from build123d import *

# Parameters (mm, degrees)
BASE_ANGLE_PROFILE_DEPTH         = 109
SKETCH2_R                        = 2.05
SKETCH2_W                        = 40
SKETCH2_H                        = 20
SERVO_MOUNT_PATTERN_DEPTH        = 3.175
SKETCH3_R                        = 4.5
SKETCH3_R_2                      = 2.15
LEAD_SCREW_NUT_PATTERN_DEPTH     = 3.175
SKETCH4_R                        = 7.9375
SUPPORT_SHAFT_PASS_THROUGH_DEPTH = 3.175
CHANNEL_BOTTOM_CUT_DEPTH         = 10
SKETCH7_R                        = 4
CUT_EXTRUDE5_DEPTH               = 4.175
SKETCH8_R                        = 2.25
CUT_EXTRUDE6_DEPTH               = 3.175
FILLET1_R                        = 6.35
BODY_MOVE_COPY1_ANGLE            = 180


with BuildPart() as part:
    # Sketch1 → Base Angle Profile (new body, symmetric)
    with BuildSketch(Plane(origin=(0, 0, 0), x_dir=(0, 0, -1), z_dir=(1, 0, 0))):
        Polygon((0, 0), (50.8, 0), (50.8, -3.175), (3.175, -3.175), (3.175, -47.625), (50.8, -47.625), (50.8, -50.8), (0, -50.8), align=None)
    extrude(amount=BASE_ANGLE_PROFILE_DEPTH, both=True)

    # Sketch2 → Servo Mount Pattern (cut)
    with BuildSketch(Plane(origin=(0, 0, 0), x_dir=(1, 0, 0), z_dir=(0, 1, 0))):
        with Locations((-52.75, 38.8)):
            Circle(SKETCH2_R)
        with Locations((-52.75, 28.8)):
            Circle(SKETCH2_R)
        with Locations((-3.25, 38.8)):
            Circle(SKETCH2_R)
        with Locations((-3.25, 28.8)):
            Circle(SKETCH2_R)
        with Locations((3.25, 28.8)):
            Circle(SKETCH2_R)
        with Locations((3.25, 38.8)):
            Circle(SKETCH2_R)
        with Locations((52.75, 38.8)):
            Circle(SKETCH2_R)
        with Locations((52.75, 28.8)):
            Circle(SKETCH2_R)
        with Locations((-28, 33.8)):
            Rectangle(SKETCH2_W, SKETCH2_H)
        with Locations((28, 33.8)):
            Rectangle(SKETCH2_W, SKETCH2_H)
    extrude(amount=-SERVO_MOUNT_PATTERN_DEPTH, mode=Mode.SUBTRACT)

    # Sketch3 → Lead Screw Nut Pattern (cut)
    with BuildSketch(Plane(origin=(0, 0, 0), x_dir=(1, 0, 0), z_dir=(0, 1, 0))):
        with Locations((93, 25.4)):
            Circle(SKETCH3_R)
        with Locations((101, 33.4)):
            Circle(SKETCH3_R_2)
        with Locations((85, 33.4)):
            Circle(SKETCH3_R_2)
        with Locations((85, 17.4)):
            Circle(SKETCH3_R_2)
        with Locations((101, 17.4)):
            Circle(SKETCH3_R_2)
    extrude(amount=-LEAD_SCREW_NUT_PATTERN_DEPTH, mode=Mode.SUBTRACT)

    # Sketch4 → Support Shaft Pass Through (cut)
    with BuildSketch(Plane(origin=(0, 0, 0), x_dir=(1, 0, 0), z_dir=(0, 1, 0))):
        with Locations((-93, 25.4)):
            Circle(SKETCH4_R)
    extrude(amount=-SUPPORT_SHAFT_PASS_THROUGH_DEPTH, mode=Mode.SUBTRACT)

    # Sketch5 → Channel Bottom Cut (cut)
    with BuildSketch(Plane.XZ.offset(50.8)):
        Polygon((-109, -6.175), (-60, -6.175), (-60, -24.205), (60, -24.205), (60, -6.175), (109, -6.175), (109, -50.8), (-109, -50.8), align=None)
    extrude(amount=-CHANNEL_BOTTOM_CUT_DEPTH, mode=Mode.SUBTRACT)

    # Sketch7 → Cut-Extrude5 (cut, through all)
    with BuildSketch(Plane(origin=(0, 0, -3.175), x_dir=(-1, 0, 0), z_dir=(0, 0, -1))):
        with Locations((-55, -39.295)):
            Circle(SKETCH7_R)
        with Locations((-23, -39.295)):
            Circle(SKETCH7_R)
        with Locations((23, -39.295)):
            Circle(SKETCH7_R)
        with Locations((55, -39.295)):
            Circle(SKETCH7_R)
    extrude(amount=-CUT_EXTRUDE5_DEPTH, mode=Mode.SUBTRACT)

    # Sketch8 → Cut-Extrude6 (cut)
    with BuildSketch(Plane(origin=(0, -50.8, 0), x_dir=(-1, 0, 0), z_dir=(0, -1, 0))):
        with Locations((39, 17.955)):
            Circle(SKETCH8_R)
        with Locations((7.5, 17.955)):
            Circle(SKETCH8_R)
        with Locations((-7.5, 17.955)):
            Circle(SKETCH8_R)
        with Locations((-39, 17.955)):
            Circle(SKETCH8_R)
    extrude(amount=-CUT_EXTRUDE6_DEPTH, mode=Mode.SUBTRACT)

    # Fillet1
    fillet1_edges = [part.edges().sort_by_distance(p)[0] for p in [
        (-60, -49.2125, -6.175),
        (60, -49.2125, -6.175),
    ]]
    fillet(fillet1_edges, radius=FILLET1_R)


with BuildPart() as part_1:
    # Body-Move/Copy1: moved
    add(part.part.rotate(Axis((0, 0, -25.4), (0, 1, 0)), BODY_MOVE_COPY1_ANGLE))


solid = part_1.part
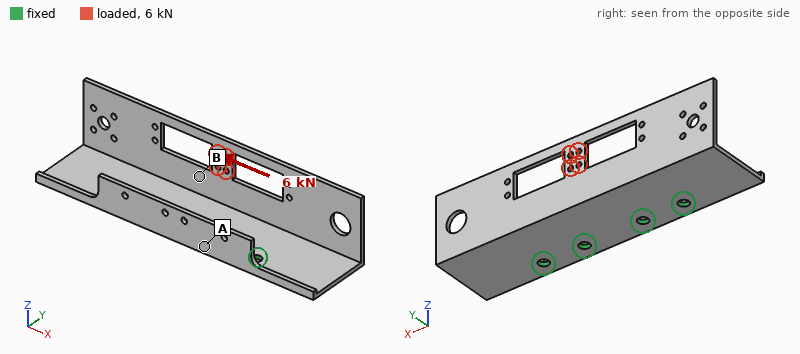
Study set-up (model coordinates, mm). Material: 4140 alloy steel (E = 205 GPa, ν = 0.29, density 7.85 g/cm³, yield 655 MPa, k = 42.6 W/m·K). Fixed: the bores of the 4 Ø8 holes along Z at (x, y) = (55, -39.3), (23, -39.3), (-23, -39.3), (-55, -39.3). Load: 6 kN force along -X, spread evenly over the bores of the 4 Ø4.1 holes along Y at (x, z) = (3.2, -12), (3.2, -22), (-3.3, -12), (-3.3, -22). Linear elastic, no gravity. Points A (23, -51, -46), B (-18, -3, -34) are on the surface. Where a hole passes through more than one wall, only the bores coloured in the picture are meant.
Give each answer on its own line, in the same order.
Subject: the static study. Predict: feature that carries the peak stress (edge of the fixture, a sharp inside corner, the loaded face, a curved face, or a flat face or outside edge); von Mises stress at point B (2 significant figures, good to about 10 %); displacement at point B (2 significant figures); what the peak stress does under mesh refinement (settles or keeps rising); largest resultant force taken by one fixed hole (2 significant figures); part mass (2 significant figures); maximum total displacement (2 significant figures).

edge of the fixture
180 MPa
0.23 mm
keeps rising
2.7 kN
550 g
1.4 mm
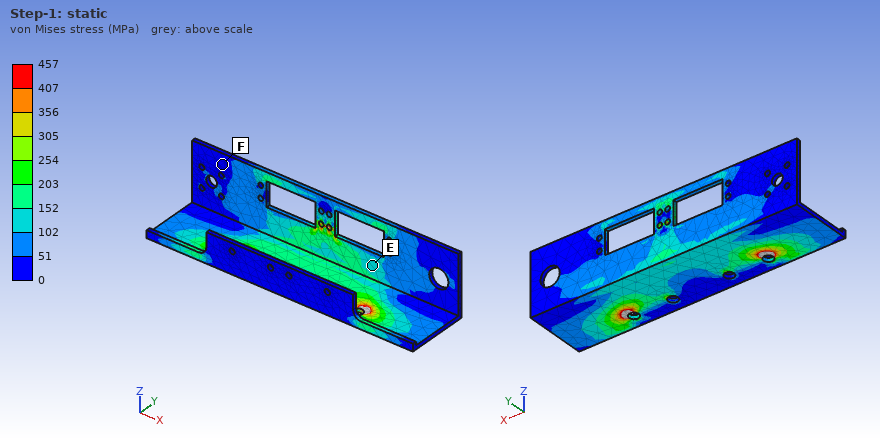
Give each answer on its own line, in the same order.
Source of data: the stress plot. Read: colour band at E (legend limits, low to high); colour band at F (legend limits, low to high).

102 to 152 MPa
0 to 51 MPa
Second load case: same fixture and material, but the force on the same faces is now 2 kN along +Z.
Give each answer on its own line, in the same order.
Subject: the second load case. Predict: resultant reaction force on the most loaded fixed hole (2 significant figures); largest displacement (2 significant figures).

770 N
0.74 mm
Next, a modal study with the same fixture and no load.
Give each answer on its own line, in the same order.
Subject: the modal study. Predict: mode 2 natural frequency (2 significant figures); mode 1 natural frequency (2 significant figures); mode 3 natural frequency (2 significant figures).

520 Hz
500 Hz
1000 Hz
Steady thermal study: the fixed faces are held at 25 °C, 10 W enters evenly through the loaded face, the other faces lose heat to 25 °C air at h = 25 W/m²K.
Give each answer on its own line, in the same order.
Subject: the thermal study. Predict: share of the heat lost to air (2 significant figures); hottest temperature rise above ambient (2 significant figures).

67 %
67 K
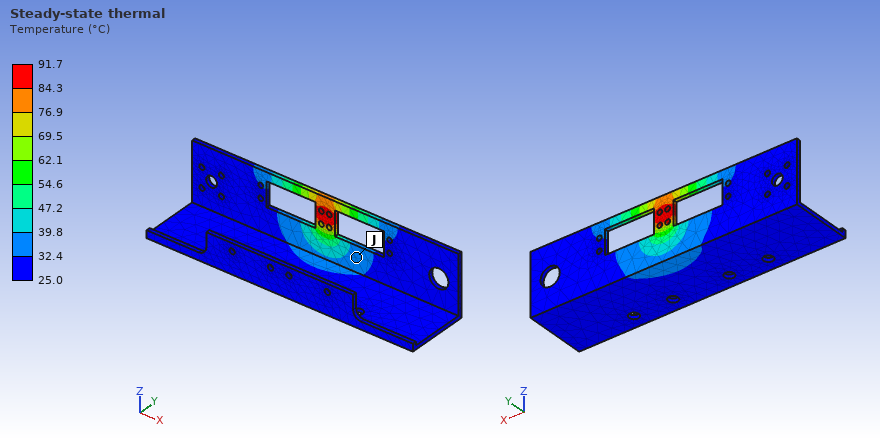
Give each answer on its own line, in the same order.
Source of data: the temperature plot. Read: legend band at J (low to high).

32.4 to 39.8 °C
